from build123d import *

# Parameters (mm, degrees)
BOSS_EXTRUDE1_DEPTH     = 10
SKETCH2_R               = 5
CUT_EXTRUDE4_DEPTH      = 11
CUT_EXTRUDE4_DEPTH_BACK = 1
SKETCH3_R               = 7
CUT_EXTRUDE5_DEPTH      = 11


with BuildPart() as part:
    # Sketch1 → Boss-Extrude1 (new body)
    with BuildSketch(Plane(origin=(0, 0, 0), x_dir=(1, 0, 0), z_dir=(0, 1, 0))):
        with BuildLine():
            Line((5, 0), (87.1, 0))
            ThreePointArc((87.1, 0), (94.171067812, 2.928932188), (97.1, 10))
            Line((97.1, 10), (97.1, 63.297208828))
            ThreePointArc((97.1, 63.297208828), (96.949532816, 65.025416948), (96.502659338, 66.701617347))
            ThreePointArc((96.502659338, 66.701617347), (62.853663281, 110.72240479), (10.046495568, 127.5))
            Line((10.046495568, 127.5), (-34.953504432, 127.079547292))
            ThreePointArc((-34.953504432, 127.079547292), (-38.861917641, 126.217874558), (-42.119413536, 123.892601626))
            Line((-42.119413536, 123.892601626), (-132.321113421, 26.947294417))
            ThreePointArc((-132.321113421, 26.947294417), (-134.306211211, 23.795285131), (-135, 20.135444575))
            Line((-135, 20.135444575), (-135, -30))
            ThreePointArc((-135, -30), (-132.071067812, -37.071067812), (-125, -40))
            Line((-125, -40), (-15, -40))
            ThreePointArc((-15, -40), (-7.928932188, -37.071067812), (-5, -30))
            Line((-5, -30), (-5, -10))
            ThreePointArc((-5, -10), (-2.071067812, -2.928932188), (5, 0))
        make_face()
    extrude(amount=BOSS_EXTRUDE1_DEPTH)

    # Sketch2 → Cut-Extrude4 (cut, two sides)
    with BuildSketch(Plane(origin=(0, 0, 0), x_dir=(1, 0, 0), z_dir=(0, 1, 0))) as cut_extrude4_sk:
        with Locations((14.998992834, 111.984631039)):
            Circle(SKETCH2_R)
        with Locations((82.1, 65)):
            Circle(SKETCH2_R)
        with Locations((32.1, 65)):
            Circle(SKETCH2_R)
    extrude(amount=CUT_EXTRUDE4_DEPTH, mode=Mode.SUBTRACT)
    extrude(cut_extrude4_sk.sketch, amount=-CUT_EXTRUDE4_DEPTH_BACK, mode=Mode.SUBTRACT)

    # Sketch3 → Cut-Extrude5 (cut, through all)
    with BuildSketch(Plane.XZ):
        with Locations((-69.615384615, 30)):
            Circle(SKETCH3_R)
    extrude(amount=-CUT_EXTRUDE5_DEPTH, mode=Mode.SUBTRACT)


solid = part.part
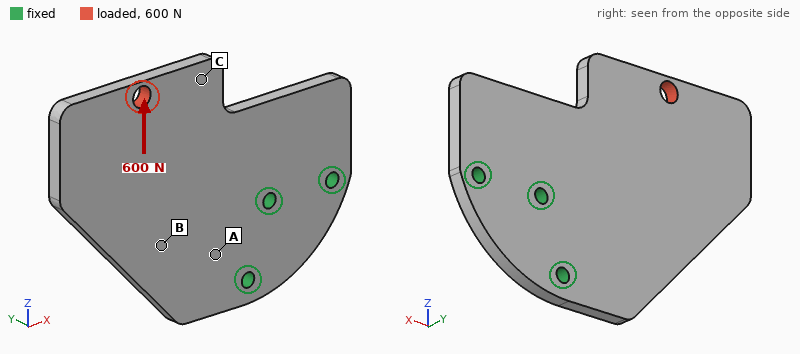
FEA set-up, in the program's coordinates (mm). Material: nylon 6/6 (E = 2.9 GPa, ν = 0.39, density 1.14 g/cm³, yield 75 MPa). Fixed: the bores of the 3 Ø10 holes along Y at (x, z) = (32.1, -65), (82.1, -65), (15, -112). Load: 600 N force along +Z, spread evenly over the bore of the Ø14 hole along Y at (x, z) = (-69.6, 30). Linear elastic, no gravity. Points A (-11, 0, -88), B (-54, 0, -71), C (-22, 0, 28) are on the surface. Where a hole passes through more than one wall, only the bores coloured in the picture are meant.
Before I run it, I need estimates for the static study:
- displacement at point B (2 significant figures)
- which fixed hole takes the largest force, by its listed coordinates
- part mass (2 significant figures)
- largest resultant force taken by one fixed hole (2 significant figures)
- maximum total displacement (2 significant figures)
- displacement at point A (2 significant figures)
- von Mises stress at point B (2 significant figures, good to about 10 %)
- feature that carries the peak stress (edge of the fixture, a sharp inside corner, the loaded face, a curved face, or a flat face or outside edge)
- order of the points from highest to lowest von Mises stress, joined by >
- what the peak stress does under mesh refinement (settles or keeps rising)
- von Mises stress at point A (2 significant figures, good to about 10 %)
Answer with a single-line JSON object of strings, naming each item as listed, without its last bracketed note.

{"displacement at point B": "0.099 mm", "which fixed hole takes the largest force, by its listed coordinates": "(15, -112)", "part mass": "320 g", "largest resultant force taken by one fixed hole": "840 N", "maximum total displacement": "0.24 mm", "displacement at point A": "0.038 mm", "von Mises stress at point B": "0.92 MPa", "feature that carries the peak stress": "edge of the fixture", "order of the points from highest to lowest von Mises stress, joined by >": "A > B > C", "what the peak stress does under mesh refinement": "keeps rising", "von Mises stress at point A": "1.7 MPa"}
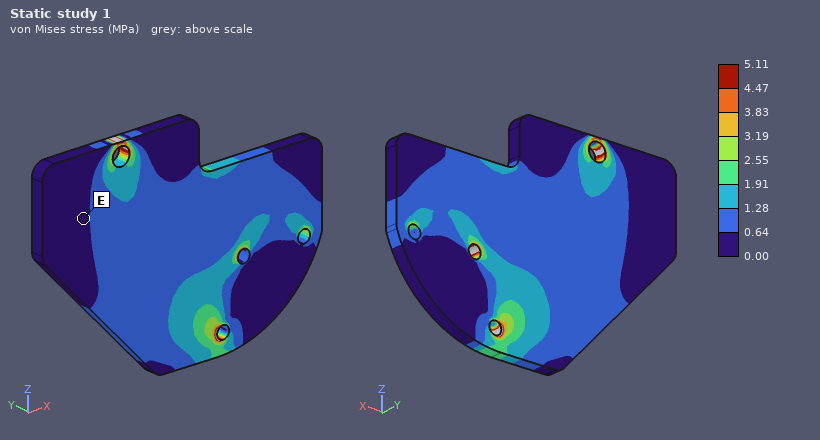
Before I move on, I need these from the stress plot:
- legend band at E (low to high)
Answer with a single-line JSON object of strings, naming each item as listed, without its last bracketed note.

{"legend band at E": "0.00 to 0.64 MPa"}
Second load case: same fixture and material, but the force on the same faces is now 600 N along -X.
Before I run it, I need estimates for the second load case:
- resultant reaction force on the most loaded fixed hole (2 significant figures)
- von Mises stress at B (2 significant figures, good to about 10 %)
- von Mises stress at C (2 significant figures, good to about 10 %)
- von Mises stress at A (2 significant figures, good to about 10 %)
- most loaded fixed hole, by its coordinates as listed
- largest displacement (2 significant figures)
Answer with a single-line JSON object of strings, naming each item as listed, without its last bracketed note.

{"resultant reaction force on the most loaded fixed hole": "760 N", "von Mises stress at B": "0.71 MPa", "von Mises stress at C": "0.64 MPa", "von Mises stress at A": "1.2 MPa", "most loaded fixed hole, by its coordinates as listed": "(32.1, -65)", "largest displacement": "0.31 mm"}
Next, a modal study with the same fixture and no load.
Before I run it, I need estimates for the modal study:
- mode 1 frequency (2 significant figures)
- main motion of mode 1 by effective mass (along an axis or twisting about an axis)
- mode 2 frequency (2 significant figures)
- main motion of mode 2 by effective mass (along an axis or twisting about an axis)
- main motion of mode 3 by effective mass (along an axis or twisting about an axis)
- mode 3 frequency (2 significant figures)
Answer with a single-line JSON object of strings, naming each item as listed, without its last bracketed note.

{"mode 1 frequency": "92 Hz", "main motion of mode 1 by effective mass": "along Y", "mode 2 frequency": "290 Hz", "main motion of mode 2 by effective mass": "twisting about X", "main motion of mode 3 by effective mass": "along Y", "mode 3 frequency": "450 Hz"}
